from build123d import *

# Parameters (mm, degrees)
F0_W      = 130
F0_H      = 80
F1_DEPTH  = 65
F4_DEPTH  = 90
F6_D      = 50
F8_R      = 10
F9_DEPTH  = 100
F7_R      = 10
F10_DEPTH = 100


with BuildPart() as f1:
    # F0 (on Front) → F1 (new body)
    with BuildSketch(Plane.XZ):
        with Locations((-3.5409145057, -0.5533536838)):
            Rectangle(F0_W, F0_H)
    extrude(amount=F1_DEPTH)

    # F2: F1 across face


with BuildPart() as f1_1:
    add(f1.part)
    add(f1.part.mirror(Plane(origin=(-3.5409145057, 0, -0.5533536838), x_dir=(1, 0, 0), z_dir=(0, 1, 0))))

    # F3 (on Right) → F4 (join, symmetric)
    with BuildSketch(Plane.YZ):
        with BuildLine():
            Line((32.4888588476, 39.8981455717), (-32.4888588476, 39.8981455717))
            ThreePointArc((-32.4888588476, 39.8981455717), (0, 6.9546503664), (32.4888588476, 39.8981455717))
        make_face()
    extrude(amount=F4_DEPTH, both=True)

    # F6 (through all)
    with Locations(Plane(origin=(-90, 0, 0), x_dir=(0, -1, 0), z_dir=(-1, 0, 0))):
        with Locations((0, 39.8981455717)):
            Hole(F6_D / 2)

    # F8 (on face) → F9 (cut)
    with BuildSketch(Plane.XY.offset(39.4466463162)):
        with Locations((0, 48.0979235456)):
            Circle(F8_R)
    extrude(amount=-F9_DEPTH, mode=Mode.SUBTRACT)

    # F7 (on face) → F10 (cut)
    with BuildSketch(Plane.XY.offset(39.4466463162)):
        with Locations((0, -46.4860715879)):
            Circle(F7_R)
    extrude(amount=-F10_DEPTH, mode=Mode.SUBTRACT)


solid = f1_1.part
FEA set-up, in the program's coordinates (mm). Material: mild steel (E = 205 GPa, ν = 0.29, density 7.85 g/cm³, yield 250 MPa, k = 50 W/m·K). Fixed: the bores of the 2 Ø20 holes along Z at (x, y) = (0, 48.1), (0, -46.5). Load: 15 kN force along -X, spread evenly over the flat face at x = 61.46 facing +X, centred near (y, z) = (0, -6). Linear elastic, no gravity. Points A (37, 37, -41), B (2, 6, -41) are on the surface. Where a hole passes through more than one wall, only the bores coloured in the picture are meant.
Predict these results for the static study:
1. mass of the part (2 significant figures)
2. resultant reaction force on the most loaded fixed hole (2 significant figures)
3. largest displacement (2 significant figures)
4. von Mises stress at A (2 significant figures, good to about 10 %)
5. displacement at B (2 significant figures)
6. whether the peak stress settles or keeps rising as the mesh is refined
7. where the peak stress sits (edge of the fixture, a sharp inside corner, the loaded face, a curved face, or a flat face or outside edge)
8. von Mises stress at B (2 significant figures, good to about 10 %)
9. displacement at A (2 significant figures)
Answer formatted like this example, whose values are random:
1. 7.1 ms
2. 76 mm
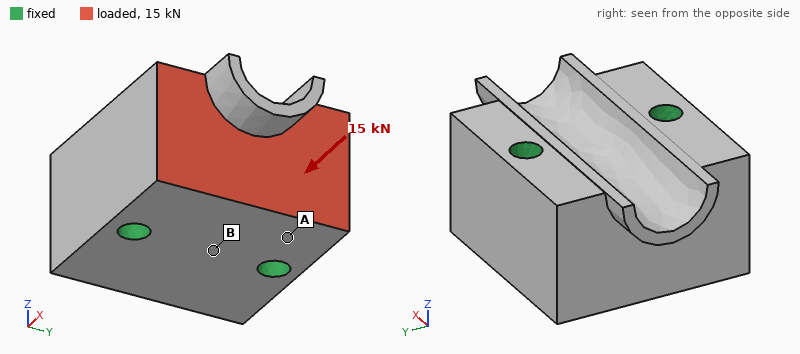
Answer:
1. 9.5 kg
2. 7.6 kN
3. 0.71 µm
4. 2.0 MPa
5. 0.30 µm
6. keeps rising
7. edge of the fixture
8. 0.80 MPa
9. 0.41 µm
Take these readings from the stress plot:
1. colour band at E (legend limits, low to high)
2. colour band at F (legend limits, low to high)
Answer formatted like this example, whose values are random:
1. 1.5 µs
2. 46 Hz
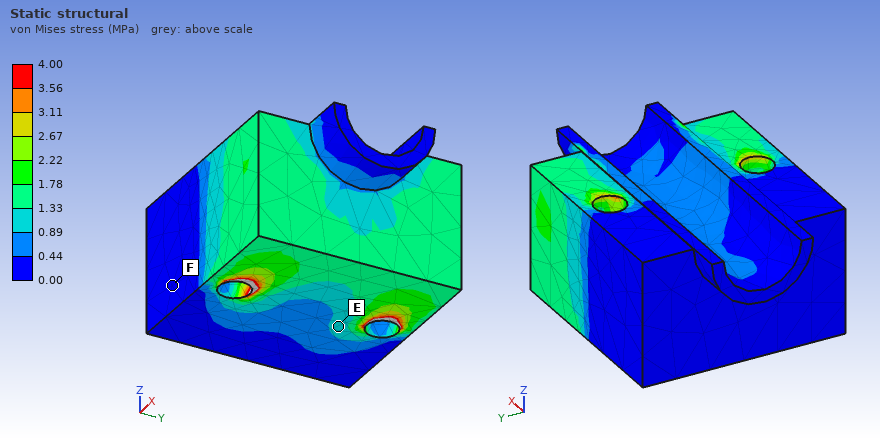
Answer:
1. 0.89 to 1.33 MPa
2. 0.00 to 0.44 MPa
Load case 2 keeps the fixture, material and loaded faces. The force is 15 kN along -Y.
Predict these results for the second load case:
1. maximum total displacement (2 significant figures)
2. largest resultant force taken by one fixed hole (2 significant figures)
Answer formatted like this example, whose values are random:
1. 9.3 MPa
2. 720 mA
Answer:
1. 2.7 µm
2. 11 kN
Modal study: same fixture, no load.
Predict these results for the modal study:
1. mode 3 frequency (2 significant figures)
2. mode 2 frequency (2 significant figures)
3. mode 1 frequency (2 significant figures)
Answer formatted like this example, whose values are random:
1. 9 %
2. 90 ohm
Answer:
1. 8500 Hz
2. 8300 Hz
3. 7600 Hz
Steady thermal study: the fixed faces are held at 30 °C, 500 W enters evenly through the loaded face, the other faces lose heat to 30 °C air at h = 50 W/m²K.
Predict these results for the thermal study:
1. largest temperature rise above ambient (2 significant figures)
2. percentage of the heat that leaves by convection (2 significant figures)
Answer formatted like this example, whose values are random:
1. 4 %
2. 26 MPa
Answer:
1. 64 K
2. 12 %
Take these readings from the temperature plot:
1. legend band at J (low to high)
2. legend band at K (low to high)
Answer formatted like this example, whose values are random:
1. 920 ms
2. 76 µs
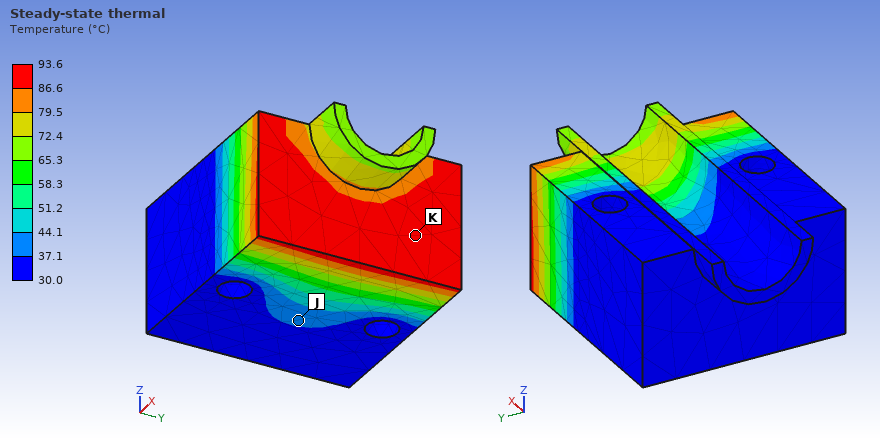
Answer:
1. 37.1 to 44.1 °C
2. 86.6 to 93.6 °C
